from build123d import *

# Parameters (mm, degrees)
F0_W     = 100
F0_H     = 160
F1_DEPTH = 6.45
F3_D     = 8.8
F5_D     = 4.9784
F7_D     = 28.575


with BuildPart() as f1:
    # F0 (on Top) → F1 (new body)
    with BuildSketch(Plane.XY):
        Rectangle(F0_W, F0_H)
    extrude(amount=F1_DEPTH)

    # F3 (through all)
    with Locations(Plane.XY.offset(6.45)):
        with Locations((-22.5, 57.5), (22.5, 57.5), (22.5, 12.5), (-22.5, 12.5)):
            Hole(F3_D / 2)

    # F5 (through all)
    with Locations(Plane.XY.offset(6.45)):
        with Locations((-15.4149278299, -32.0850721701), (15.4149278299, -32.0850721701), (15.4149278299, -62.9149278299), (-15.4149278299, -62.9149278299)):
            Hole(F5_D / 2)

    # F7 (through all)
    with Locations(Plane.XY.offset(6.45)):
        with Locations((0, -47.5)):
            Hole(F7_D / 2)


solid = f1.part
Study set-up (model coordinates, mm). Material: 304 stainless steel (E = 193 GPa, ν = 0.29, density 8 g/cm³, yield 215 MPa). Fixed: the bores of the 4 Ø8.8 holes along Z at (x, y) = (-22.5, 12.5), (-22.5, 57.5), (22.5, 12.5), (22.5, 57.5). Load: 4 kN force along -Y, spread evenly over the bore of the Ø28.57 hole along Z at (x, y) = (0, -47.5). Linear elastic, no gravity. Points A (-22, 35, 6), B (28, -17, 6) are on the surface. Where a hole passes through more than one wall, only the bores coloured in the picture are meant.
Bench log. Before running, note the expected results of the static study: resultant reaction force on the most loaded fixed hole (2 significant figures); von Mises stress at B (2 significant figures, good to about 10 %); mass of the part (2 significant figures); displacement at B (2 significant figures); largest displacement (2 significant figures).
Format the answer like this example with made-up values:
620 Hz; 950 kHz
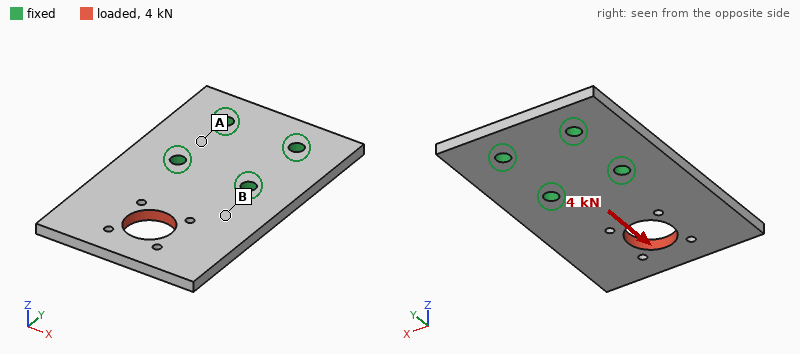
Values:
1.7 kN; 8.1 MPa; 780 g; 1.4 µm; 5.0 µm
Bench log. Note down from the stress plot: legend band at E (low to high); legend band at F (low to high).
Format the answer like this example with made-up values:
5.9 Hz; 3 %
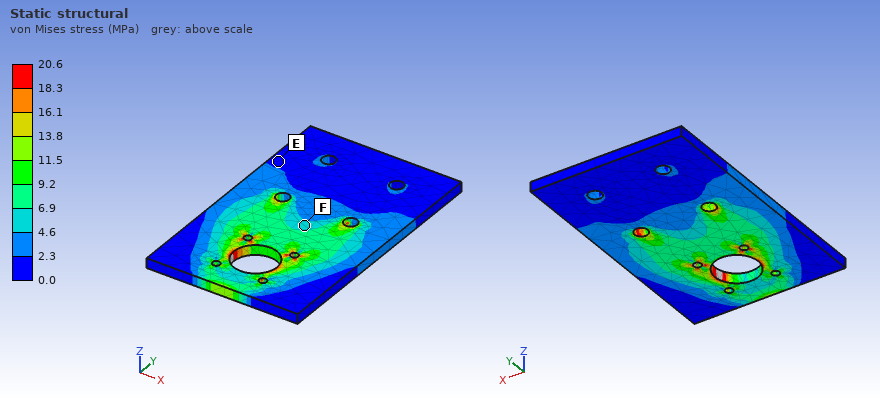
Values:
0.0 to 2.3 MPa; 4.6 to 6.9 MPa
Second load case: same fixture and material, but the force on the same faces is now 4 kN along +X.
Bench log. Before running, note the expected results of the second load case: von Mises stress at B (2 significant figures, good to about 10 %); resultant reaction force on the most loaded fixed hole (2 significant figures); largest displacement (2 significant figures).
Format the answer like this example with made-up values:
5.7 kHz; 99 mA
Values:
10 MPa; 3.8 kN; 20 µm
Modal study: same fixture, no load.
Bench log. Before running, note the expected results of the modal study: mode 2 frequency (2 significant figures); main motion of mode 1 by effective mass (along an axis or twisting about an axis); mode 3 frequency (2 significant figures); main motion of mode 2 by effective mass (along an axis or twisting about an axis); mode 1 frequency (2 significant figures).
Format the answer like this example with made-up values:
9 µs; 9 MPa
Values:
1200 Hz; along Z; 3200 Hz; twisting about Y; 630 Hz
